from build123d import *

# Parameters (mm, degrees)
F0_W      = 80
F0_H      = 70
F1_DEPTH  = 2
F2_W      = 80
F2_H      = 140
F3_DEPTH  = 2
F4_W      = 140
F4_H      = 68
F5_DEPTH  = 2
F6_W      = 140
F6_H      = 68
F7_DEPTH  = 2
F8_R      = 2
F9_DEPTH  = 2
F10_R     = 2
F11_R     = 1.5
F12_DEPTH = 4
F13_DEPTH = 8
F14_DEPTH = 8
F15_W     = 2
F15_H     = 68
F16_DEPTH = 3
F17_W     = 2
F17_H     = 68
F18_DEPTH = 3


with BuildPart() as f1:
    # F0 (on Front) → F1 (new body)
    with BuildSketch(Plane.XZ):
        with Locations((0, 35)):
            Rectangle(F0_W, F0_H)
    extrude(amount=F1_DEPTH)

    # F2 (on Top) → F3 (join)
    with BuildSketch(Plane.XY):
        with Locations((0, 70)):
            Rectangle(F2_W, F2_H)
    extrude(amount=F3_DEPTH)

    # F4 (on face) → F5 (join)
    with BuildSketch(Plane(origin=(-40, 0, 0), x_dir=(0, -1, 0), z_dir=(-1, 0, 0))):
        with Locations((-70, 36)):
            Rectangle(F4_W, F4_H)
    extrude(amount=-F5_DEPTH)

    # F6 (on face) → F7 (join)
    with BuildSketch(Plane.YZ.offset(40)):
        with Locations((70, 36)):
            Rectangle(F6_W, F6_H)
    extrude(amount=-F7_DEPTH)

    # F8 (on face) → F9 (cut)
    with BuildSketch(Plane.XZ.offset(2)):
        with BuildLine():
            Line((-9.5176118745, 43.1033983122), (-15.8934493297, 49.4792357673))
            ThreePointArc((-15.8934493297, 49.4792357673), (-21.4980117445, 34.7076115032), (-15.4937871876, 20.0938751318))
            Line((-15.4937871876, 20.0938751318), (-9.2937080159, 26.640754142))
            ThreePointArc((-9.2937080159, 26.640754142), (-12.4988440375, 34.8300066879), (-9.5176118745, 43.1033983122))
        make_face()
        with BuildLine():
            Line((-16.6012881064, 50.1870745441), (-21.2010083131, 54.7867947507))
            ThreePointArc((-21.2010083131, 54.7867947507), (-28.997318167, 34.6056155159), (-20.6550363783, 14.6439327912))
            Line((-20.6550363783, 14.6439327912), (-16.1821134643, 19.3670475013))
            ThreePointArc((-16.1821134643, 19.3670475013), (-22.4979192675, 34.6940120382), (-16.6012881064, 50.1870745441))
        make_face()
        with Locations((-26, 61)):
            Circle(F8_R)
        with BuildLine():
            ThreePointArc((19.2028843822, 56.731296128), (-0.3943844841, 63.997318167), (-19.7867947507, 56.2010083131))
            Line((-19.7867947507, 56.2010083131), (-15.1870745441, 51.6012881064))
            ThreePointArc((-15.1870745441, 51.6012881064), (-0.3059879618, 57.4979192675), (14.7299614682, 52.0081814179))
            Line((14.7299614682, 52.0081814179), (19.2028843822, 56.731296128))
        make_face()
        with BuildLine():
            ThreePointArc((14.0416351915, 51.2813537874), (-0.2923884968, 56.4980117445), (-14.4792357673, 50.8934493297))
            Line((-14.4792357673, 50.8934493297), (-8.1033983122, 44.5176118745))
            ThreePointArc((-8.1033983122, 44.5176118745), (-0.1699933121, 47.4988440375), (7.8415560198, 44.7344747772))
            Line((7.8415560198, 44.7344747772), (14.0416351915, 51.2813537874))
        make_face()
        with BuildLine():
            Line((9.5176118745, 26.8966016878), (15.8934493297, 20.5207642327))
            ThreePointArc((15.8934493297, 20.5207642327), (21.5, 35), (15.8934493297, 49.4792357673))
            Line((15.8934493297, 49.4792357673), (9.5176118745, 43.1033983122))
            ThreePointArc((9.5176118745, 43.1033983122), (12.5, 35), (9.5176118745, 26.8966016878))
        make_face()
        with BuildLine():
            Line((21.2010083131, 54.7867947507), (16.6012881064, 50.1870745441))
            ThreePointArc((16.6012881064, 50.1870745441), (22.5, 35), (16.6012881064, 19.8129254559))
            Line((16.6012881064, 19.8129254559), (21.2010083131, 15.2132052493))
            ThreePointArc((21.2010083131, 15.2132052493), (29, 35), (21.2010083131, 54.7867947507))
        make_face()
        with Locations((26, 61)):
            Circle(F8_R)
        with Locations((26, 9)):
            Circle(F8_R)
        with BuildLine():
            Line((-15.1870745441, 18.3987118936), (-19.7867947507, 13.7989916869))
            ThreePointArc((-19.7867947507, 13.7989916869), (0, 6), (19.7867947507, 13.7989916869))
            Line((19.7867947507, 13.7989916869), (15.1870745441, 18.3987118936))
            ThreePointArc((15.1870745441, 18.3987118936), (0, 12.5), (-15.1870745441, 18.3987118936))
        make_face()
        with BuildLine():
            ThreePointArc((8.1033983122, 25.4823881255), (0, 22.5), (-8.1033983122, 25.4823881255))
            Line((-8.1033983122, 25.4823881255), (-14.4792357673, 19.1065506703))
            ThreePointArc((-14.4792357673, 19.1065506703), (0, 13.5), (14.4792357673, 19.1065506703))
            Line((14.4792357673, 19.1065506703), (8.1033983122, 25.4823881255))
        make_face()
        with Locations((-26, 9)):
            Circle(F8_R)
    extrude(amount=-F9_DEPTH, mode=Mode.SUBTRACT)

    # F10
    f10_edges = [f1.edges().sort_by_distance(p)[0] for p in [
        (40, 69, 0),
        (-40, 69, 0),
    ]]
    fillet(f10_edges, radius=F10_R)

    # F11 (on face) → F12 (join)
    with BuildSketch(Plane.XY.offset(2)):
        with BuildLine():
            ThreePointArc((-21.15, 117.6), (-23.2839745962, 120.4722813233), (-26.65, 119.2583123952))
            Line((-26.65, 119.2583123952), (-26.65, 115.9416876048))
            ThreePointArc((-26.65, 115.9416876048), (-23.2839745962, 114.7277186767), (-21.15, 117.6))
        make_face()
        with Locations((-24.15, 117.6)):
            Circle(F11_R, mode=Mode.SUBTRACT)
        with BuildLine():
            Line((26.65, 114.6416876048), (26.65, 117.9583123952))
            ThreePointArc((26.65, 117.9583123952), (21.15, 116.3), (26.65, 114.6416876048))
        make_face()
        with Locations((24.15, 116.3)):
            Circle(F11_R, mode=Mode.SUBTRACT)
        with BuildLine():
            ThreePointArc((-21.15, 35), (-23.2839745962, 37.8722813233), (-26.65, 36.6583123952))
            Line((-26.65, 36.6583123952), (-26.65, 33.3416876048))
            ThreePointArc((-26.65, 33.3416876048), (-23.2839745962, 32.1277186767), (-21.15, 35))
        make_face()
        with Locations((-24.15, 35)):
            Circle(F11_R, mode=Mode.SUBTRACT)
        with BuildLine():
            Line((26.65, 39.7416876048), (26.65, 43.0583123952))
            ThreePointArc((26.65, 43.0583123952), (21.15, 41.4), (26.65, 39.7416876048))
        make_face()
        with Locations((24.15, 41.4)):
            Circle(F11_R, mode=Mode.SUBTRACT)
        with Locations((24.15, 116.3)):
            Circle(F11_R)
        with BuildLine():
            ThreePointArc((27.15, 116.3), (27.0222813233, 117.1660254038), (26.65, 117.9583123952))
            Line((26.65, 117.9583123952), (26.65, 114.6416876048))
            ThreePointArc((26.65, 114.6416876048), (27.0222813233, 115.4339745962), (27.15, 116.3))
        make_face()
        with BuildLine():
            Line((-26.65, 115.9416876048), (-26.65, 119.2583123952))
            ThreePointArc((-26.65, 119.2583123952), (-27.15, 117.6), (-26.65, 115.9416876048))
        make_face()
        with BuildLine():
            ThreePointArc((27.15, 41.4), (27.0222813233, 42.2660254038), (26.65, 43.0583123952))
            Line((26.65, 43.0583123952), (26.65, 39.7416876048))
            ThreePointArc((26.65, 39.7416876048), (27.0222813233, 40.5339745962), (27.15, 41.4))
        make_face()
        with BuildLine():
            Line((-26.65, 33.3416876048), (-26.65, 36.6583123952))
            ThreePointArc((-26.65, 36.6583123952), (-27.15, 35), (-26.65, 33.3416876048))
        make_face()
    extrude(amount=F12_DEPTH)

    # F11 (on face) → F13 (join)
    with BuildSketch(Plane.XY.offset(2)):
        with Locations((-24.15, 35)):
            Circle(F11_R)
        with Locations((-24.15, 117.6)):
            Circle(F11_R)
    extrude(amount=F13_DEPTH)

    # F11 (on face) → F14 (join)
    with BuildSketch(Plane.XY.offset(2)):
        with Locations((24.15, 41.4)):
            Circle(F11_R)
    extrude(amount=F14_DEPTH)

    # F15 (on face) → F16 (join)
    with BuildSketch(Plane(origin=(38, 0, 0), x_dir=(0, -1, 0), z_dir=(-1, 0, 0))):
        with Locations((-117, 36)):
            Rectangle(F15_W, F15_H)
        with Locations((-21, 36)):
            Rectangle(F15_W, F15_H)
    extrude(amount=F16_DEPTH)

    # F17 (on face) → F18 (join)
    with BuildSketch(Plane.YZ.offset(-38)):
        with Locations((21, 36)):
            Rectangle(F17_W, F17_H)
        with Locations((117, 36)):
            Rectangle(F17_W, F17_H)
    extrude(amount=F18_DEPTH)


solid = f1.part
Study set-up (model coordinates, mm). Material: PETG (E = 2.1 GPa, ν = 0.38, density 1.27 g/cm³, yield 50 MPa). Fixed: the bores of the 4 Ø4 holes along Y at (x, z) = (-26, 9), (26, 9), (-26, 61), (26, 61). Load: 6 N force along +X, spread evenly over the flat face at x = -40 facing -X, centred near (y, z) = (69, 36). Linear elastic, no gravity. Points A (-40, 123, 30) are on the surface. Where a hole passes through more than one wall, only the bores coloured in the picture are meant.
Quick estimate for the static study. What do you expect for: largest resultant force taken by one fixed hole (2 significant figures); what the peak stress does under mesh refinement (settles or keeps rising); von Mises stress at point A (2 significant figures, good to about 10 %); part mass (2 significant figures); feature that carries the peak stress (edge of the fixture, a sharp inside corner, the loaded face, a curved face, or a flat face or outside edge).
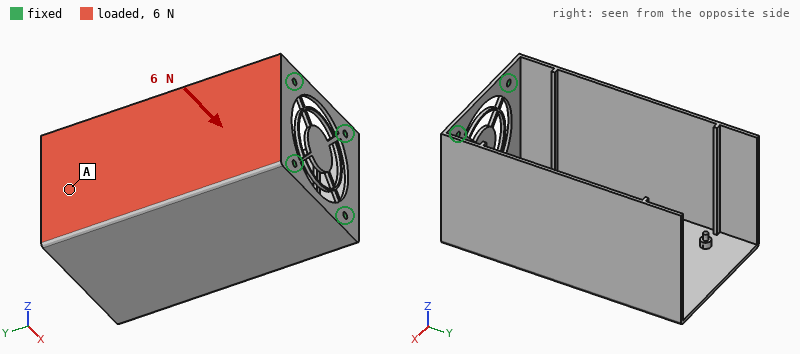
10 N
keeps rising
0.34 MPa
89 g
edge of the fixture
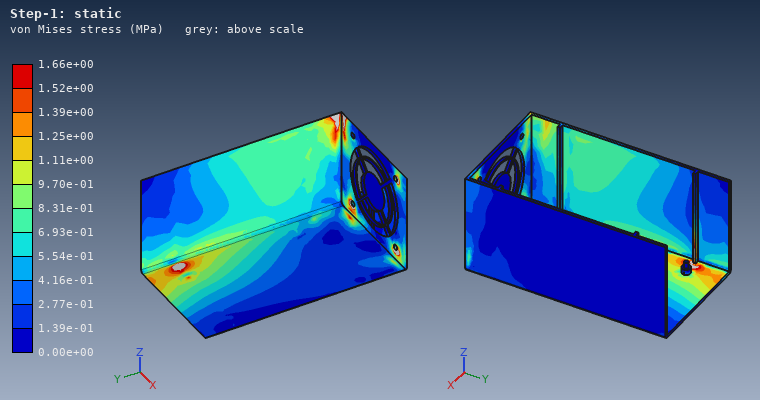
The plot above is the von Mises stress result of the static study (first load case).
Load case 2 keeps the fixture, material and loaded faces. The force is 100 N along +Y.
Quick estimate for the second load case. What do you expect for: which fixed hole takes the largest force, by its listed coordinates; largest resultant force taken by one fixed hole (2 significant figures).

(-26, 9)
65 N
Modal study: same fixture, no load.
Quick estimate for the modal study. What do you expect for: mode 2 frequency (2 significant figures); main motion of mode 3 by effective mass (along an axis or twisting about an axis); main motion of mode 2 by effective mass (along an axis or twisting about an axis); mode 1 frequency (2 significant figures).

79 Hz
along Z
along X
72 Hz
